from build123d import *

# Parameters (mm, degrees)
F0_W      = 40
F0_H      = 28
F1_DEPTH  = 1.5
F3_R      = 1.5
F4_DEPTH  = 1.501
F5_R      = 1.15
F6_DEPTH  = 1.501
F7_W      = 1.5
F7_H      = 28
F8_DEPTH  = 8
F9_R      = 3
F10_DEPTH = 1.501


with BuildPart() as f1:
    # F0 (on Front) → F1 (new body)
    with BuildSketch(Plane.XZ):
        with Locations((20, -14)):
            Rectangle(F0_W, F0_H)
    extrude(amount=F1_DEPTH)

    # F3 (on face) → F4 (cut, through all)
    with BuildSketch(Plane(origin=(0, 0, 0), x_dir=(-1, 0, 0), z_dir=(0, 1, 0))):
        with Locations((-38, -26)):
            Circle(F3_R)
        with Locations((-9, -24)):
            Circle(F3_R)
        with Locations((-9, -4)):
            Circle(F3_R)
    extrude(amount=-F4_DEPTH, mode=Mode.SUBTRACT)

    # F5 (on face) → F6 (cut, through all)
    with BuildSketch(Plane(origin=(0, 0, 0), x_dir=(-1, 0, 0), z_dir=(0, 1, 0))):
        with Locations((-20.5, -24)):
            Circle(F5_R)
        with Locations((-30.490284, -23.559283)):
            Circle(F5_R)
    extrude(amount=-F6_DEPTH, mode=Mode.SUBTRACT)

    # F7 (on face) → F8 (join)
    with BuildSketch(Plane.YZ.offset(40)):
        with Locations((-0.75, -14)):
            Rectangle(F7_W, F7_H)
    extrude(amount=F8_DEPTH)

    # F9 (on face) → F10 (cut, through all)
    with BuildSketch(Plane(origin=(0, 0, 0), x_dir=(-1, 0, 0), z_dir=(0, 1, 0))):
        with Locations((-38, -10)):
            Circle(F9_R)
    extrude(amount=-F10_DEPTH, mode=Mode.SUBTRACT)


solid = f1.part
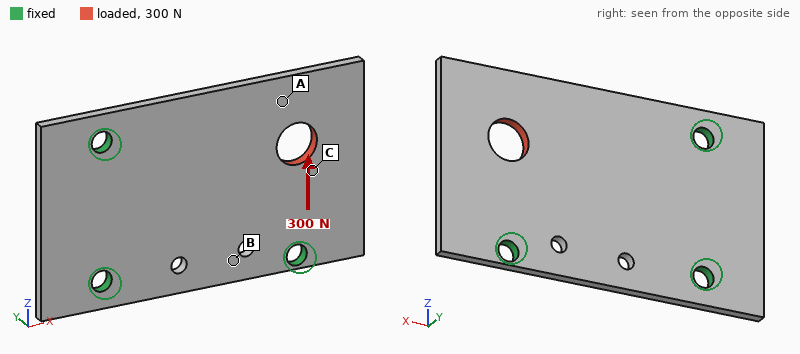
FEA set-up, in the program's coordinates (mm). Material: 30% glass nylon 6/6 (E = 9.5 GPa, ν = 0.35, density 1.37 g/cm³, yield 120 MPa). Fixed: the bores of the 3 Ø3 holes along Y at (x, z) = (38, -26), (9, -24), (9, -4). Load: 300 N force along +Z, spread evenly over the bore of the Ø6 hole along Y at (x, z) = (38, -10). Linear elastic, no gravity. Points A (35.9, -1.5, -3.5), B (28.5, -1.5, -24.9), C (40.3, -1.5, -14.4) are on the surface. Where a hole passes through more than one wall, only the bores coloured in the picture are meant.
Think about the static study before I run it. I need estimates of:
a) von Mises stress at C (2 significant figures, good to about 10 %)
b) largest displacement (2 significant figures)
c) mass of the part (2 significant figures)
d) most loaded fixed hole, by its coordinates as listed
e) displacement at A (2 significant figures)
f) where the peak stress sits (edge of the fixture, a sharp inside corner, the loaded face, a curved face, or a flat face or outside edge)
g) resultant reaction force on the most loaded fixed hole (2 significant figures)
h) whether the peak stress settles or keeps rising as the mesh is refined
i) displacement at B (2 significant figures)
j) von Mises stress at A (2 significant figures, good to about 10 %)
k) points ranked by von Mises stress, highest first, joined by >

17 MPa
37 µm
2.6 g
(38, -26)
31 µm
edge of the fixture
250 N
keeps rising
11 µm
7.5 MPa
C > A > B
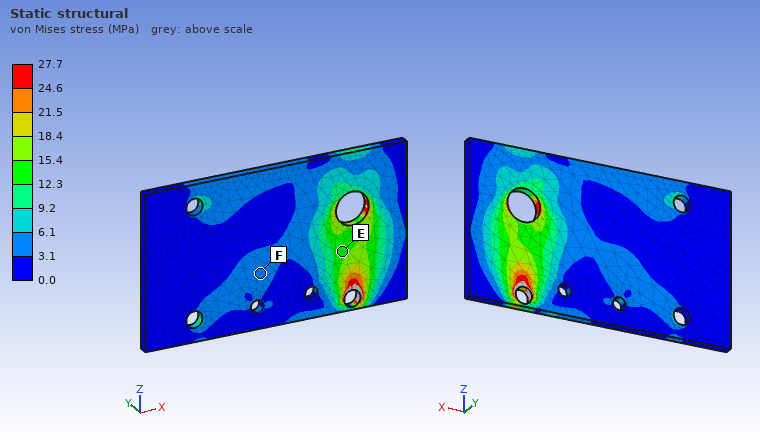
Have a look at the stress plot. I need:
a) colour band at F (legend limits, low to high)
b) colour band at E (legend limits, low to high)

3.1 to 6.1 MPa
12.3 to 15.4 MPa
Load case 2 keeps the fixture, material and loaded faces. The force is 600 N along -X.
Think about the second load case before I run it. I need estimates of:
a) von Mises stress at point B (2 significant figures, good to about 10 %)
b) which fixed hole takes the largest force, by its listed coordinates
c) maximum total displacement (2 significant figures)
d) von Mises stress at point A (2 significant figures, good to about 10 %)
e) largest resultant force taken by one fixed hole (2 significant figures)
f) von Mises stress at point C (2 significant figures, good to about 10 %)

6.6 MPa
(9, -4)
76 µm
18 MPa
290 N
15 MPa
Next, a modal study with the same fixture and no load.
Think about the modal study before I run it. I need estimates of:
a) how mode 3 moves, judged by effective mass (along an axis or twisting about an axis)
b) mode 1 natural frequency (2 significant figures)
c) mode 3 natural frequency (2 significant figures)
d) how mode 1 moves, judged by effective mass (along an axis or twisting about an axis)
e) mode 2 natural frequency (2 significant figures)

along Y
1300 Hz
5000 Hz
along Y
3200 Hz
